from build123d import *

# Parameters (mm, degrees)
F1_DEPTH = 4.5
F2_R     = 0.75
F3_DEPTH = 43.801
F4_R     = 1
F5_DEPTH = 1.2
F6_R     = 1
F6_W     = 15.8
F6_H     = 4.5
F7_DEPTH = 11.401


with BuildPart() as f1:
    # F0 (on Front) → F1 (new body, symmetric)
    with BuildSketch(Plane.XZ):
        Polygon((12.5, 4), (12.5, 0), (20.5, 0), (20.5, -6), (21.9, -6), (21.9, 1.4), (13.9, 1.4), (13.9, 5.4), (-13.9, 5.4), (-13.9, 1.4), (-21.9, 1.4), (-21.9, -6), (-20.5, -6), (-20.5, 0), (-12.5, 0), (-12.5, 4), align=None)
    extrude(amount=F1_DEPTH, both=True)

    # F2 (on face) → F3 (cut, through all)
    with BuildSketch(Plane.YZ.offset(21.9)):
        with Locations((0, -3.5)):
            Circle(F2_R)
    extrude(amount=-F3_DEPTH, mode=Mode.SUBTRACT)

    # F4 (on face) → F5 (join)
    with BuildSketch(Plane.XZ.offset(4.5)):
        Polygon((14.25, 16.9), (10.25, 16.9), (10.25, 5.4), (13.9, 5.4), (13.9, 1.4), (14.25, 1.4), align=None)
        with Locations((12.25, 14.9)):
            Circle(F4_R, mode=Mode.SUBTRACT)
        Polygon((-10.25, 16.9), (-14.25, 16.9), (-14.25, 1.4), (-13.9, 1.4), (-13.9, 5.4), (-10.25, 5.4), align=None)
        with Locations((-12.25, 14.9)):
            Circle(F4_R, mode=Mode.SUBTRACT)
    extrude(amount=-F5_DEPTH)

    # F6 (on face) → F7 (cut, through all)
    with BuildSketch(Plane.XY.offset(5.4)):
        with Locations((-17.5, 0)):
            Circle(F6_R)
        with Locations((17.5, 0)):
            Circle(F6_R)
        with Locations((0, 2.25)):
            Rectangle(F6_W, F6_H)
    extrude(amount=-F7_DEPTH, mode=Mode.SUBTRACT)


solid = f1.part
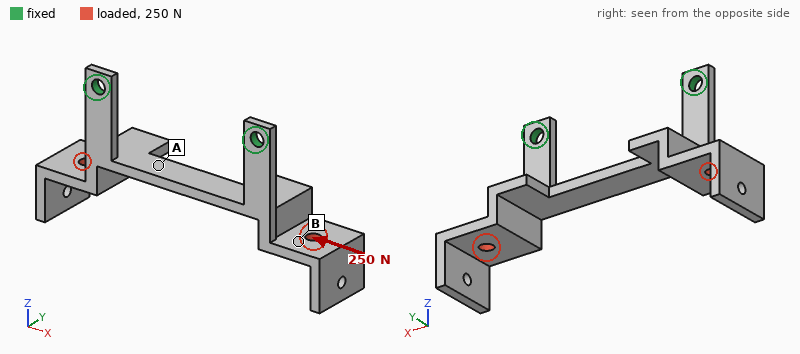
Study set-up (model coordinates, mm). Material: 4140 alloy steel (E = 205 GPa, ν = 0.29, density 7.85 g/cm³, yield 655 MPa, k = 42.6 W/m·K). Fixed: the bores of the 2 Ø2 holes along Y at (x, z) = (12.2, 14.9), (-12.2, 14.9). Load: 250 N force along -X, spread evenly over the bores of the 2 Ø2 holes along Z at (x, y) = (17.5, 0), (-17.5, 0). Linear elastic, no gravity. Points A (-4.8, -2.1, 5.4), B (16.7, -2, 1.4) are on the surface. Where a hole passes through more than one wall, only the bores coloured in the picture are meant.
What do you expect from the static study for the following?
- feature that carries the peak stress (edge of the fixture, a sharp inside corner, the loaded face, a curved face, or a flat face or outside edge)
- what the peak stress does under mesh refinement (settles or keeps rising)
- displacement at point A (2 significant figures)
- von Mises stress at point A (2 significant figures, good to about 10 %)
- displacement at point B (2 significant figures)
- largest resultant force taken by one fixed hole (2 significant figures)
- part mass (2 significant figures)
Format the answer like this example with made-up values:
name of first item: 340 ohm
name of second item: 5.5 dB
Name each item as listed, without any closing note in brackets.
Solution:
feature that carries the peak stress: edge of the fixture
what the peak stress does under mesh refinement: keeps rising
displacement at point A: 0.053 mm
von Mises stress at point A: 140 MPa
displacement at point B: 0.095 mm
largest resultant force taken by one fixed hole: 140 N
part mass: 6.3 g
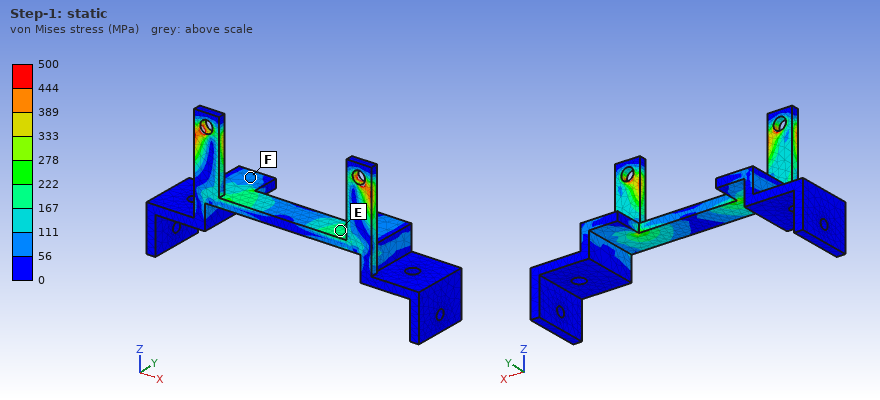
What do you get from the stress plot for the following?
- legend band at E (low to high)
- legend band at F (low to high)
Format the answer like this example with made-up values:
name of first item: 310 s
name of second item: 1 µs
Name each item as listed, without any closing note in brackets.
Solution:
legend band at E: 167 to 222 MPa
legend band at F: 56 to 111 MPa
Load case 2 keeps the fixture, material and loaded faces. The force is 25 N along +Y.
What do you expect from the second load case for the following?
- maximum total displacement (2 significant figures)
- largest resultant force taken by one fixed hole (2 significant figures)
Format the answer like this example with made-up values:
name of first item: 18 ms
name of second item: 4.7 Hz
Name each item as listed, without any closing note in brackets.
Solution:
maximum total displacement: 0.16 mm
largest resultant force taken by one fixed hole: 13 N
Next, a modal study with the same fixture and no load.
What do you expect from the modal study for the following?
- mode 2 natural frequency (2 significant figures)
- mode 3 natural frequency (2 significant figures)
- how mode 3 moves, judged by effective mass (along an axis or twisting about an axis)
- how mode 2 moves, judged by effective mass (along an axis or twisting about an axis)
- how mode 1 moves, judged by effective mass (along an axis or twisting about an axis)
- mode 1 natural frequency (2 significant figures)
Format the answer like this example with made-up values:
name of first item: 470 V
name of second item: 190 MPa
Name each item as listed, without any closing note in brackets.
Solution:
mode 2 natural frequency: 1600 Hz
mode 3 natural frequency: 3000 Hz
how mode 3 moves, judged by effective mass: along X
how mode 2 moves, judged by effective mass: twisting about Z
how mode 1 moves, judged by effective mass: along Y
mode 1 natural frequency: 1100 Hz
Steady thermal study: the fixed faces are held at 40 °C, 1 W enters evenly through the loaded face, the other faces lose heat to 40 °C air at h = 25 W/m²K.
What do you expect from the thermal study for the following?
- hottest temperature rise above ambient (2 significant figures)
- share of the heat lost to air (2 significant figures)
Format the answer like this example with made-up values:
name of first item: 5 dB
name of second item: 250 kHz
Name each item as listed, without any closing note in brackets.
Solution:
hottest temperature rise above ambient: 19 K
share of the heat lost to air: 49 %
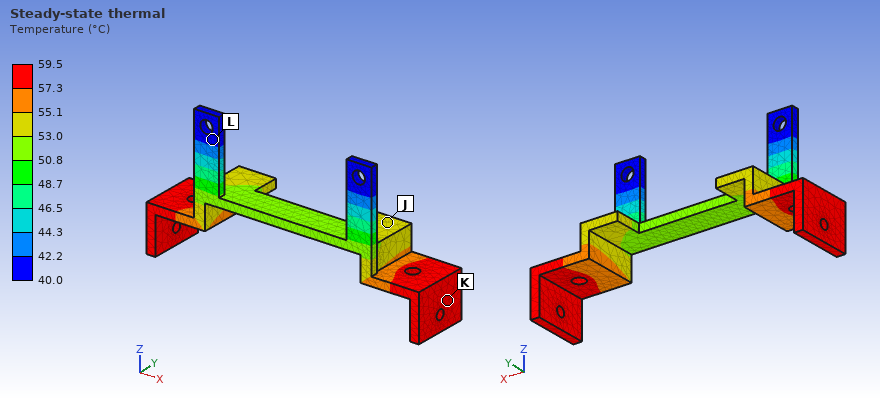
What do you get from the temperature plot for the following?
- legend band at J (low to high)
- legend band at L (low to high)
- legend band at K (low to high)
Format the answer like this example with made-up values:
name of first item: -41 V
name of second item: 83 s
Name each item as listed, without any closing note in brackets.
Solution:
legend band at J: 53.0 to 55.1 °C
legend band at L: 40.0 to 42.2 °C
legend band at K: 57.3 to 59.5 °C
